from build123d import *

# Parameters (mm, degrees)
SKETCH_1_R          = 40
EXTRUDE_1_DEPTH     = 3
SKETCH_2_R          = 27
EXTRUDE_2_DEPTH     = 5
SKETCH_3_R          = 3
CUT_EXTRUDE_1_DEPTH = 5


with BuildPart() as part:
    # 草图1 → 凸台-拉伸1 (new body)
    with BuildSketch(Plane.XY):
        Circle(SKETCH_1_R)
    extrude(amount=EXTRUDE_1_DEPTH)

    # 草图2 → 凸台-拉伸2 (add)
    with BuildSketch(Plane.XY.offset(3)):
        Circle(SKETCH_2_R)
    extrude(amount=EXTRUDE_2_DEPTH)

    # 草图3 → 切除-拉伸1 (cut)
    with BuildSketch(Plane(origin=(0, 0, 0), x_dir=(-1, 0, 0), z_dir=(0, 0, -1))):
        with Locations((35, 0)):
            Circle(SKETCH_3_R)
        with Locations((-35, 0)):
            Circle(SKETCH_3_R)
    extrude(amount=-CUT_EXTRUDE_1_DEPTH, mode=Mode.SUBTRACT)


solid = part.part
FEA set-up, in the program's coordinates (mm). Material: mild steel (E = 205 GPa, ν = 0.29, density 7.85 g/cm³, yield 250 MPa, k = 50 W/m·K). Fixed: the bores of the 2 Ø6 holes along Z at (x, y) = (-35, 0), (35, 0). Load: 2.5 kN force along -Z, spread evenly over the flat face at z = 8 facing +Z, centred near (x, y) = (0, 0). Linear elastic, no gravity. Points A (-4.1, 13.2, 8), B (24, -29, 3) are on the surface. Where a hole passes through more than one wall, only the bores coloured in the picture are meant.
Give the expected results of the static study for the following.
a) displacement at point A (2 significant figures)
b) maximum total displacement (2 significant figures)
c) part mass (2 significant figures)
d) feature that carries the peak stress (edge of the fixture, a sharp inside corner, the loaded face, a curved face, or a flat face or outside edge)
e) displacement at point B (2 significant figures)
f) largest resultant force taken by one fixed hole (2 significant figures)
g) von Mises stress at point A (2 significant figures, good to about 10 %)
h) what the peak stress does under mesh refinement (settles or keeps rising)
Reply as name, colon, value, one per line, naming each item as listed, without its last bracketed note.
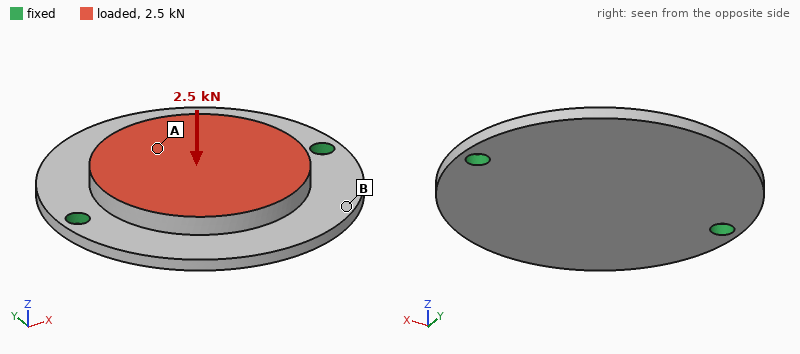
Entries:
displacement at point A: 27 µm
maximum total displacement: 38 µm
part mass: 210 g
feature that carries the peak stress: edge of the fixture
displacement at point B: 24 µm
largest resultant force taken by one fixed hole: 2.1 kN
von Mises stress at point A: 36 MPa
what the peak stress does under mesh refinement: keeps rising
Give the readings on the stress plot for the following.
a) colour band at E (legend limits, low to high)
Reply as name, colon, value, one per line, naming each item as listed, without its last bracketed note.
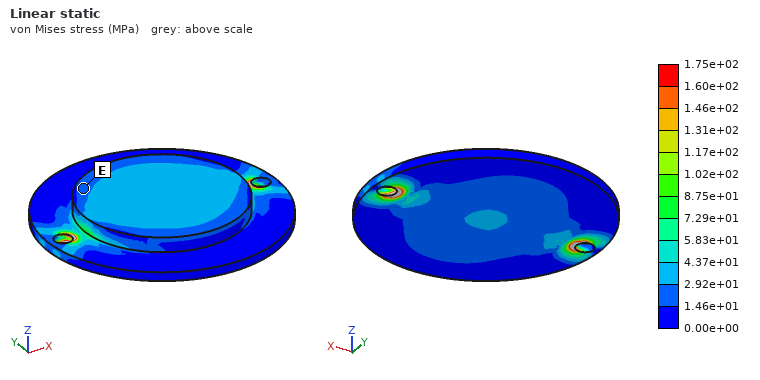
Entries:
colour band at E: 1.46e+01 to 2.92e+01 MPa
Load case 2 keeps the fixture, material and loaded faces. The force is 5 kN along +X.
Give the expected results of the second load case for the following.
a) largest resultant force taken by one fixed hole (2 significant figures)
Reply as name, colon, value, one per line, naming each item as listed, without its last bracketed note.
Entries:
largest resultant force taken by one fixed hole: 2.6 kN
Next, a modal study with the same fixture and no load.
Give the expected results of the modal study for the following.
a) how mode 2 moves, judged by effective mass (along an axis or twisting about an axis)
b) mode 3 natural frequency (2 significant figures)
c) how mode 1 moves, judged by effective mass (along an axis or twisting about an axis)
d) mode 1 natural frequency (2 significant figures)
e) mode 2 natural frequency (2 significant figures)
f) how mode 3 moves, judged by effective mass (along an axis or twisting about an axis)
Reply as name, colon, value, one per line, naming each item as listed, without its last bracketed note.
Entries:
how mode 2 moves, judged by effective mass: along Z
mode 3 natural frequency: 7400 Hz
how mode 1 moves, judged by effective mass: twisting about X
mode 1 natural frequency: 1600 Hz
mode 2 natural frequency: 3500 Hz
how mode 3 moves, judged by effective mass: twisting about Y
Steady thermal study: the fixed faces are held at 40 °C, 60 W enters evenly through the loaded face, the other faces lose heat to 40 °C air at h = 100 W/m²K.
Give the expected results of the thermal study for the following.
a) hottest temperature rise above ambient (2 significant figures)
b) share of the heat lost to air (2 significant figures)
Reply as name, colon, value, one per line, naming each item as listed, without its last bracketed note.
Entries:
hottest temperature rise above ambient: 53 K
share of the heat lost to air: 55 %
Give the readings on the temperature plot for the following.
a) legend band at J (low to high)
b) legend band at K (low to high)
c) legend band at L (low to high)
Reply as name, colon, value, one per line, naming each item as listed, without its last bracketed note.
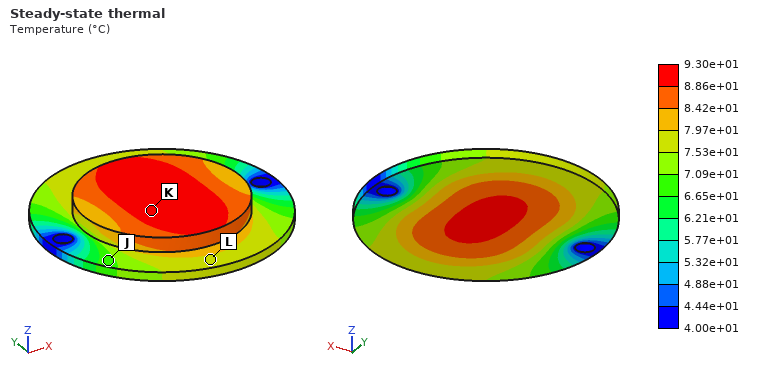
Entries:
legend band at J: 6.65e+01 to 7.09e+01 °C
legend band at K: 8.86e+01 to 9.30e+01 °C
legend band at L: 7.53e+01 to 7.97e+01 °C
